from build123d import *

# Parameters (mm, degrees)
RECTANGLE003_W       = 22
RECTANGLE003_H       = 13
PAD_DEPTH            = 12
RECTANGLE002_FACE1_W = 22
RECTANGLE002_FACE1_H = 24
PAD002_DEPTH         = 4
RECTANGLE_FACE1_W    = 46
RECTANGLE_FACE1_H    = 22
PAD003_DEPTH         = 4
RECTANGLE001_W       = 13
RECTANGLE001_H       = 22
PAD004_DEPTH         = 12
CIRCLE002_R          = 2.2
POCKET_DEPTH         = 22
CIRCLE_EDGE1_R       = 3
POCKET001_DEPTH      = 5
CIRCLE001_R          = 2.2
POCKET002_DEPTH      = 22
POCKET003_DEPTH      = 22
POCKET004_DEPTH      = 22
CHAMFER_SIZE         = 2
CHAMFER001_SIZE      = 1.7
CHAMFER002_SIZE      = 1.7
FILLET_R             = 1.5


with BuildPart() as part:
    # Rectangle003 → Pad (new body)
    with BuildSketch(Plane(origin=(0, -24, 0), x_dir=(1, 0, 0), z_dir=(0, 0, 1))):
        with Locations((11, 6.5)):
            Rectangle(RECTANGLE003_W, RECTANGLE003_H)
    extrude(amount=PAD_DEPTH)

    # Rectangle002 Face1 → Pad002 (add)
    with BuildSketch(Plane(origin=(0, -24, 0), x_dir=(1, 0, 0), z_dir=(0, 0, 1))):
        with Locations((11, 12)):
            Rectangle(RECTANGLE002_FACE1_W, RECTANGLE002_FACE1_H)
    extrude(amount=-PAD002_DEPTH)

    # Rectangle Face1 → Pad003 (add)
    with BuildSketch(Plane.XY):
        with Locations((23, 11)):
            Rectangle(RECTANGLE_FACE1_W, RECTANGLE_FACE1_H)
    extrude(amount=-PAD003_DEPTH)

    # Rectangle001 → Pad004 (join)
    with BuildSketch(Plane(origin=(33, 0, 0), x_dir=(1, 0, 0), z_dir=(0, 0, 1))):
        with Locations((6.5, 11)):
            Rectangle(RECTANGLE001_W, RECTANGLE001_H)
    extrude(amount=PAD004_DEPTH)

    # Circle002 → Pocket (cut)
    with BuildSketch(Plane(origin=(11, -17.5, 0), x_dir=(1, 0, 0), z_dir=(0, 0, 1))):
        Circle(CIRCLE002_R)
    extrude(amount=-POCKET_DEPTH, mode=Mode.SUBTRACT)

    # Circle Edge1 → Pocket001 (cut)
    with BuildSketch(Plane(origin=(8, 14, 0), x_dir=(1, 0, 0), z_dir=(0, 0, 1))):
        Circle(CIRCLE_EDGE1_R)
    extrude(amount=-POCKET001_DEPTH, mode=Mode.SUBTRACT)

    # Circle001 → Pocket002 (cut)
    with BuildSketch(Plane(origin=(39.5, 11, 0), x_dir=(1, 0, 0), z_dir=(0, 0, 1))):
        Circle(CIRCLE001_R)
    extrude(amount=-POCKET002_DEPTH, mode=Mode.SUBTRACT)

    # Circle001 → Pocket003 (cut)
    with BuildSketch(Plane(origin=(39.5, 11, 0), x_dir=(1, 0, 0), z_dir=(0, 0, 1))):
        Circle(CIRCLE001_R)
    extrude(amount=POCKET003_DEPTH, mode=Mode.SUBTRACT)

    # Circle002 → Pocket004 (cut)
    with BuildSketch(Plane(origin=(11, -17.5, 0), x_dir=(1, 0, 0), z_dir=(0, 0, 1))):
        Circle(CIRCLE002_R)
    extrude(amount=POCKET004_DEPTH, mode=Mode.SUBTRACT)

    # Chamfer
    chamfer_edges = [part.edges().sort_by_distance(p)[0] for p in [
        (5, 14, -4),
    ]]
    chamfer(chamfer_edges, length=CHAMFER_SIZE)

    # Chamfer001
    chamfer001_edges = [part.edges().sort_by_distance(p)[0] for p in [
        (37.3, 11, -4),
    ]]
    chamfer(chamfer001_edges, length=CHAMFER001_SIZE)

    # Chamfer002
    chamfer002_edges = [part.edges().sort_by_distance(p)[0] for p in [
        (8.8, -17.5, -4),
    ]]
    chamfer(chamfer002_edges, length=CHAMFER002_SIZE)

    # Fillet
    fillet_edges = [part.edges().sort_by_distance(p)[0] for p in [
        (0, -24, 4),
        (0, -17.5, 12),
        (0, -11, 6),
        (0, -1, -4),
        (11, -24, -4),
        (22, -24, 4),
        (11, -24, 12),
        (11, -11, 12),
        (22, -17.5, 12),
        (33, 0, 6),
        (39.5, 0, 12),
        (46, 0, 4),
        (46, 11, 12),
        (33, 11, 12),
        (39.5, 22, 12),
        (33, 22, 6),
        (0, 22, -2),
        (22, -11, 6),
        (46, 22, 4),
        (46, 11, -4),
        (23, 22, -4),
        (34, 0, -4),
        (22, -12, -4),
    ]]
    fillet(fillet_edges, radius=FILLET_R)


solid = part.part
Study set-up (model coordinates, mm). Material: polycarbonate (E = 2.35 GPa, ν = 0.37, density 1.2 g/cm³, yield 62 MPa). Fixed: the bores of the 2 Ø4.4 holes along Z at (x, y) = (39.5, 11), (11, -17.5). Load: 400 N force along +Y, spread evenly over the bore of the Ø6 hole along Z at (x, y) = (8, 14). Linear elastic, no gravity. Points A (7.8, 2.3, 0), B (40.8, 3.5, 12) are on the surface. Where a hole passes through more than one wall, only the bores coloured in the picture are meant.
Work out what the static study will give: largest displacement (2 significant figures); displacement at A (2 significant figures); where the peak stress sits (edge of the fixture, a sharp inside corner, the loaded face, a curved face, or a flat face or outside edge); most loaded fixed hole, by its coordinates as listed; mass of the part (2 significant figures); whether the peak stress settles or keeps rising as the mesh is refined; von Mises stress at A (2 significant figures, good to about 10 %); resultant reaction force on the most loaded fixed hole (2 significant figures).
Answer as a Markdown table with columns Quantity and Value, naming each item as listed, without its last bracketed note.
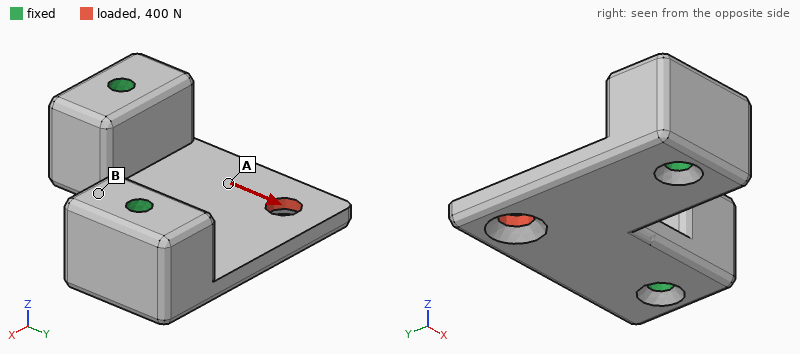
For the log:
| Quantity | Value |
|---|---|
| largest displacement | 0.32 mm |
| displacement at A | 0.059 mm |
| where the peak stress sits | a sharp inside corner |
| most loaded fixed hole, by its coordinates as listed | (11, -17.5) |
| mass of the part | 15 g |
| whether the peak stress settles or keeps rising as the mesh is refined | keeps rising |
| von Mises stress at A | 8.9 MPa |
| resultant reaction force on the most loaded fixed hole | 380 N |
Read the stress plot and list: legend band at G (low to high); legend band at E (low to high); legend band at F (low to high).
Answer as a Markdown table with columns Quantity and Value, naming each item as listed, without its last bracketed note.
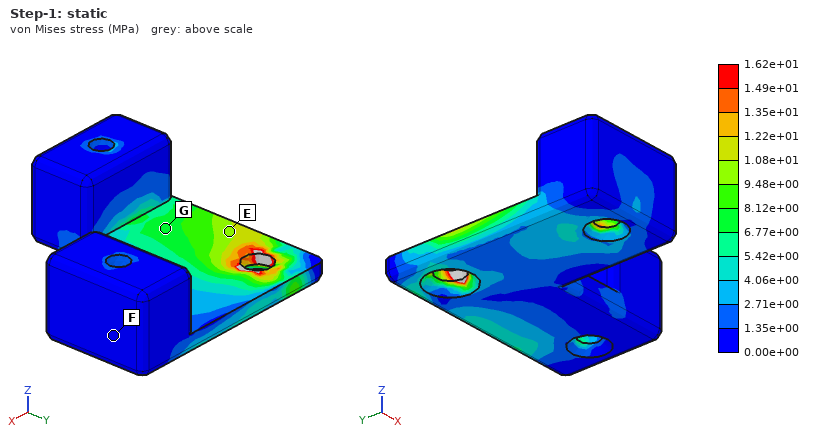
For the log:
| Quantity | Value |
|---|---|
| legend band at G | 6.77e+00 to 8.12e+00 MPa |
| legend band at E | 9.48e+00 to 1.08e+01 MPa |
| legend band at F | 0.00e+00 to 1.35e+00 MPa |
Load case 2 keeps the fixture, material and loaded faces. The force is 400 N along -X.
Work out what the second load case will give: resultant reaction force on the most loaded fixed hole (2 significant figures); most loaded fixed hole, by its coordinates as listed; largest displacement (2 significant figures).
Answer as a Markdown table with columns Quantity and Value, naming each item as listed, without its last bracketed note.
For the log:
| Quantity | Value |
|---|---|
| resultant reaction force on the most loaded fixed hole | 380 N |
| most loaded fixed hole, by its coordinates as listed | (39.5, 11) |
| largest displacement | 0.32 mm |
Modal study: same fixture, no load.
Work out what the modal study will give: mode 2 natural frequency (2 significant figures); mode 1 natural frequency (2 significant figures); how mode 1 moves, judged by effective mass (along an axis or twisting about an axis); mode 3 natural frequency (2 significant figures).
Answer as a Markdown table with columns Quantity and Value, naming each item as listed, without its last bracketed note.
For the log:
| Quantity | Value |
|---|---|
| mode 2 natural frequency | 4400 Hz |
| mode 1 natural frequency | 1500 Hz |
| how mode 1 moves, judged by effective mass | along Z |
| mode 3 natural frequency | 4900 Hz |
